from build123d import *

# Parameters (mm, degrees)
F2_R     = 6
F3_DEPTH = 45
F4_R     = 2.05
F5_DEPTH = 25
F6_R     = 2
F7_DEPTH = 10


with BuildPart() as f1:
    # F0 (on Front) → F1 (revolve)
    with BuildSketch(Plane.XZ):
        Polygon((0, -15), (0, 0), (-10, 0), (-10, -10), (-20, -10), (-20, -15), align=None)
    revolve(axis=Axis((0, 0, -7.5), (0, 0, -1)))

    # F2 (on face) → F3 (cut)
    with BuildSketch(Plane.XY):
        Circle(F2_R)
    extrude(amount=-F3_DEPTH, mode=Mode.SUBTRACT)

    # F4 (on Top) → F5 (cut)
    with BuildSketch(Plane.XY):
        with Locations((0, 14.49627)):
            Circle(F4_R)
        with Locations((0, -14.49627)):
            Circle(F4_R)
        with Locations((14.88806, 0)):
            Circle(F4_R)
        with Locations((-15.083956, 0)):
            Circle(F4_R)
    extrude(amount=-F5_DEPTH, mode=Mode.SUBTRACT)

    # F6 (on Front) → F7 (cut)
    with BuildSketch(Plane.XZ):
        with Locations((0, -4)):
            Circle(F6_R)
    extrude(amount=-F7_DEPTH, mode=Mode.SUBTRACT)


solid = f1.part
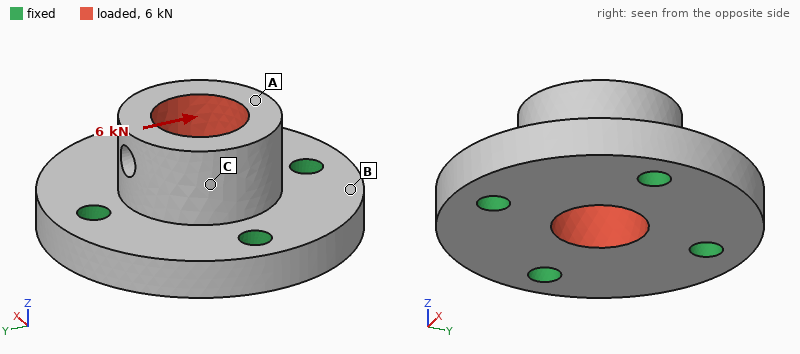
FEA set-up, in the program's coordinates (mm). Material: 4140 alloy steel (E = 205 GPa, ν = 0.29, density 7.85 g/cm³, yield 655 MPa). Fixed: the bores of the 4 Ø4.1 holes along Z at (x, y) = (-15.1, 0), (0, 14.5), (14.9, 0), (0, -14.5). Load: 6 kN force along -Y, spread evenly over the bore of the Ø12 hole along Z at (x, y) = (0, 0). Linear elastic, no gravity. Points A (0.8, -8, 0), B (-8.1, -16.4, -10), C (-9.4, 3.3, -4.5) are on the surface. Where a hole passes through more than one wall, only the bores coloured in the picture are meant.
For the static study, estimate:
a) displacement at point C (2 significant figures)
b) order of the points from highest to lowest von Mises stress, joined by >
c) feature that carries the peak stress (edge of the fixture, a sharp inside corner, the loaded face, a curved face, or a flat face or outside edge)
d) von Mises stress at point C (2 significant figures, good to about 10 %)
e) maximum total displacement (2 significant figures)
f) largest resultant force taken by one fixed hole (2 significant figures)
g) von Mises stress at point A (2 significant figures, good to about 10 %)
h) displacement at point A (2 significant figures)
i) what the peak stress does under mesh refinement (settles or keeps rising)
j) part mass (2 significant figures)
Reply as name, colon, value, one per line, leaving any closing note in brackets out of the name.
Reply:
displacement at point C: 3.9 µm
order of the points from highest to lowest von Mises stress, joined by >: A > C > B
feature that carries the peak stress: edge of the fixture
von Mises stress at point C: 18 MPa
maximum total displacement: 6.7 µm
largest resultant force taken by one fixed hole: 2.2 kN
von Mises stress at point A: 29 MPa
displacement at point A: 6.5 µm
what the peak stress does under mesh refinement: keeps rising
part mass: 58 g
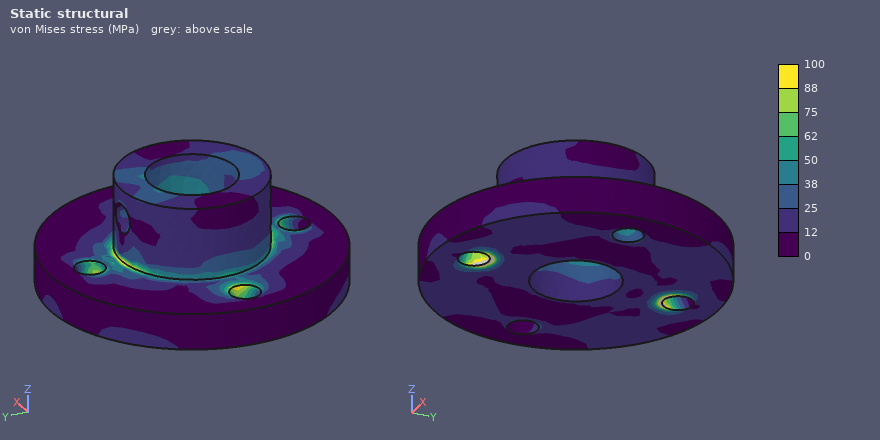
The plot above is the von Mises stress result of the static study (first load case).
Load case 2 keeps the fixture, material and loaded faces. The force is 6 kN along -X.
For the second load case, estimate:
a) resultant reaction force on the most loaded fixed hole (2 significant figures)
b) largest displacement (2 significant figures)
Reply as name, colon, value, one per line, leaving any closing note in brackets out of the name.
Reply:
resultant reaction force on the most loaded fixed hole: 2.1 kN
largest displacement: 7.1 µm
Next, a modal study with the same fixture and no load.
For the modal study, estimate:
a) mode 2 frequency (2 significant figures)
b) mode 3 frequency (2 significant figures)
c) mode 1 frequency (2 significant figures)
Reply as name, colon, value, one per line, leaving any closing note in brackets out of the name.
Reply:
mode 2 frequency: 34 kHz
mode 3 frequency: 37 kHz
mode 1 frequency: 33 kHz
